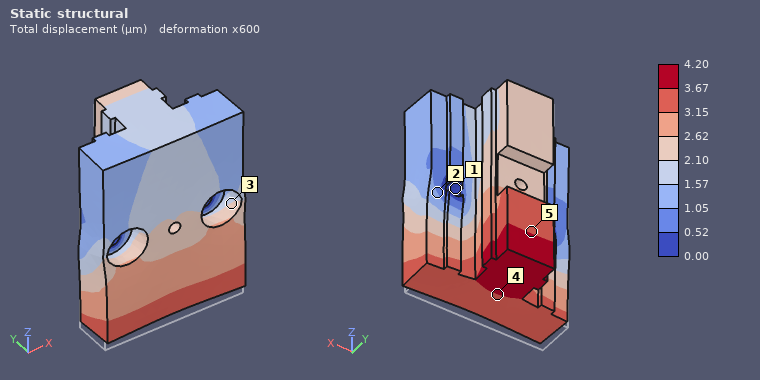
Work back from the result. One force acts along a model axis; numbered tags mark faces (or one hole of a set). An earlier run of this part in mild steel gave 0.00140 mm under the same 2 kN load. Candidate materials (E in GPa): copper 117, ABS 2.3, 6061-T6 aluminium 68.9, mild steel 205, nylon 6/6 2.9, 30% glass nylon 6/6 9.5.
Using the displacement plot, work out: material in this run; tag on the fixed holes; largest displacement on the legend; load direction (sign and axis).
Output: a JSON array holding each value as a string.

["6061-T6 aluminium", "1", "4.20 µm", "+Z"]
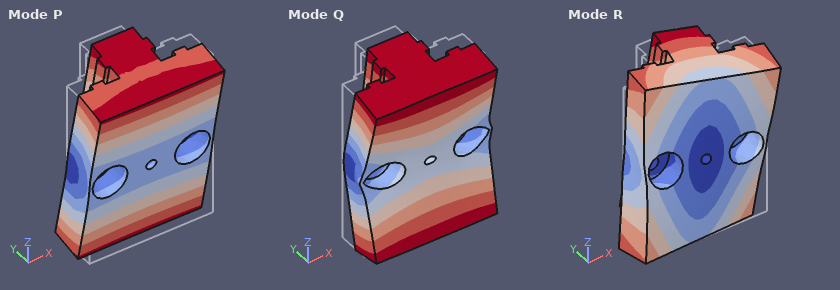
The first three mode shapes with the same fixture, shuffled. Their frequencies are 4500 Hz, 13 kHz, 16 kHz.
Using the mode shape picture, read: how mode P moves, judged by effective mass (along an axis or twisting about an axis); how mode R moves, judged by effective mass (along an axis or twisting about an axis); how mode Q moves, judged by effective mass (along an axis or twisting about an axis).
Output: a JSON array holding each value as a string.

["twisting about X", "twisting about Y", "along Y"]
